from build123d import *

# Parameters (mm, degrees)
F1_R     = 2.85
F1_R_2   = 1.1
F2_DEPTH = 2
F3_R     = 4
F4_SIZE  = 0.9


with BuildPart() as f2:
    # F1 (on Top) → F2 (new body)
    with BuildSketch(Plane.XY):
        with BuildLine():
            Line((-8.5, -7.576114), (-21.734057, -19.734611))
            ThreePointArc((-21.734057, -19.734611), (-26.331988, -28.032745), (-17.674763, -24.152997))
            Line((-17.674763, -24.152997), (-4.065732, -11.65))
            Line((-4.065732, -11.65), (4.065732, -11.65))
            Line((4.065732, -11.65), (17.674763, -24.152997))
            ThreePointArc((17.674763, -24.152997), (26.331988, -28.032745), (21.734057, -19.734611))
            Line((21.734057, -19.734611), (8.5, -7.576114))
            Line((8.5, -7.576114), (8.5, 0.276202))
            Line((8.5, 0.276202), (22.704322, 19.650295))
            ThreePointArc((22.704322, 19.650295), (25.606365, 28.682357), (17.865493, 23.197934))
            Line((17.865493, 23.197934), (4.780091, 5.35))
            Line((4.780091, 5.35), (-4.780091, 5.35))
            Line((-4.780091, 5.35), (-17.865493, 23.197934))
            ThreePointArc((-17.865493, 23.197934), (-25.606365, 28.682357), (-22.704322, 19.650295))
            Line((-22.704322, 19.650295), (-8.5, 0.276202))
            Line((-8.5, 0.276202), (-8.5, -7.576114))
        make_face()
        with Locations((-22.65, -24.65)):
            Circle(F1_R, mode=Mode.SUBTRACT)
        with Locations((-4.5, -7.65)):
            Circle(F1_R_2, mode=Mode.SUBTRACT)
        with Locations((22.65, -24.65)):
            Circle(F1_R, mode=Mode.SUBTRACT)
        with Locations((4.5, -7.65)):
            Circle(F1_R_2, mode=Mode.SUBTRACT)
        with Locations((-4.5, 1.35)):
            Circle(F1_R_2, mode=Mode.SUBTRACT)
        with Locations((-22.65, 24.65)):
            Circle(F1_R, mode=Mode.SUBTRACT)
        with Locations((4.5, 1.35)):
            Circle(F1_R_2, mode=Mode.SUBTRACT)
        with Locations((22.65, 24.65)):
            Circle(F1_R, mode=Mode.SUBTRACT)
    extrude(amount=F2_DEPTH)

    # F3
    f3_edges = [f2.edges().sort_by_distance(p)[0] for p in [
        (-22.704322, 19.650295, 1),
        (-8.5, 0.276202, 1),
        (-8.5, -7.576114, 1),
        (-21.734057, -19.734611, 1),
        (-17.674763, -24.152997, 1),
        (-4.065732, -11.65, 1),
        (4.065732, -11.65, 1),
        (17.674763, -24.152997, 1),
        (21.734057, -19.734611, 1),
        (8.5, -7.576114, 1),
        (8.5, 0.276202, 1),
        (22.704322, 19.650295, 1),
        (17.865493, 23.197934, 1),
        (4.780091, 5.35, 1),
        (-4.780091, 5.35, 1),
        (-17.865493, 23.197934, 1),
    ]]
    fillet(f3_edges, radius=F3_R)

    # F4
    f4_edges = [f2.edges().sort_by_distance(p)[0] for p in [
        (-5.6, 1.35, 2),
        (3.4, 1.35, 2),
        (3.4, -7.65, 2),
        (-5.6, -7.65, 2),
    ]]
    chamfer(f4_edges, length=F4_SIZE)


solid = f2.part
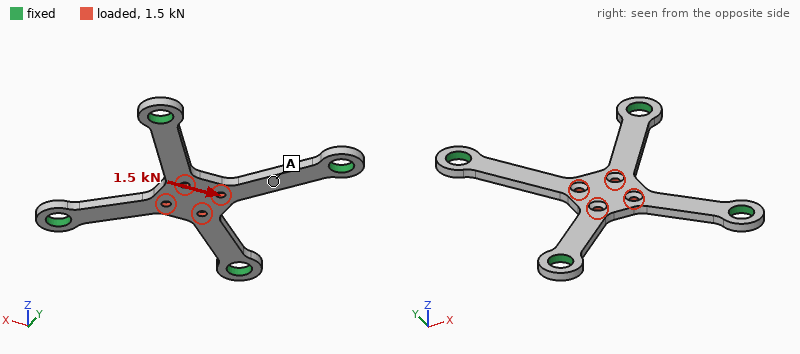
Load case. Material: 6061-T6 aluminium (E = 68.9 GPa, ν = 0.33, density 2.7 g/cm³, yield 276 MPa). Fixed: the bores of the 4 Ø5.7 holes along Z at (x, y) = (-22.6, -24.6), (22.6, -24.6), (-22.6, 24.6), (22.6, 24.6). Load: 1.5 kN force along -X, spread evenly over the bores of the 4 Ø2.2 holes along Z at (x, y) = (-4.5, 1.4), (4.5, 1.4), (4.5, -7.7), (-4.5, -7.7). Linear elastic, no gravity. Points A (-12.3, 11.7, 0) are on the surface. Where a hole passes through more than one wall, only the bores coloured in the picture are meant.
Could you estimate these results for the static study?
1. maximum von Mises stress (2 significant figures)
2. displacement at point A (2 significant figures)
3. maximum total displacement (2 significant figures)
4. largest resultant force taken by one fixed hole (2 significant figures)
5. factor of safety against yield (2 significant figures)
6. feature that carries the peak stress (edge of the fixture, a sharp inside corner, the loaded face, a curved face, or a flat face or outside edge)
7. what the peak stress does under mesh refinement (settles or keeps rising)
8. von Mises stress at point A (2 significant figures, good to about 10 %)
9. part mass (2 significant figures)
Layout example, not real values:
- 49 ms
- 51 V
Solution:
- 140 MPa
- 24 µm
- 43 µm
- 620 N
- 2.0
- the loaded face
- settles
- 48 MPa
- 5.0 g
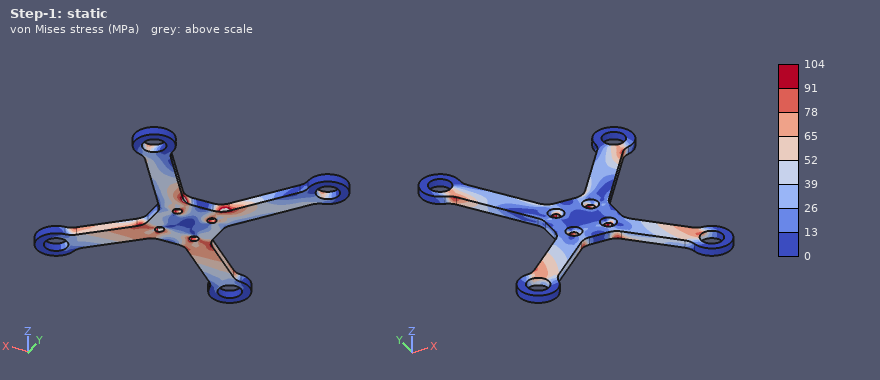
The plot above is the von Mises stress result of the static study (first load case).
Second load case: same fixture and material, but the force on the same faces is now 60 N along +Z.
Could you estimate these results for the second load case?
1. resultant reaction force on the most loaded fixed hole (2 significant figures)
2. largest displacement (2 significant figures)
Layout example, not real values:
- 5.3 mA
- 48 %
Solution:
- 18 N
- 87 µm
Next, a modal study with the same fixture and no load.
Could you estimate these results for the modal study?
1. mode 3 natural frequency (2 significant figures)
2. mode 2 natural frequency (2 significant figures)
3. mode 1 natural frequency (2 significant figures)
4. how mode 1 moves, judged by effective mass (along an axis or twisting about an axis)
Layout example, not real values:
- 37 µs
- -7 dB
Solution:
- 7800 Hz
- 7300 Hz
- 3000 Hz
- along Z
